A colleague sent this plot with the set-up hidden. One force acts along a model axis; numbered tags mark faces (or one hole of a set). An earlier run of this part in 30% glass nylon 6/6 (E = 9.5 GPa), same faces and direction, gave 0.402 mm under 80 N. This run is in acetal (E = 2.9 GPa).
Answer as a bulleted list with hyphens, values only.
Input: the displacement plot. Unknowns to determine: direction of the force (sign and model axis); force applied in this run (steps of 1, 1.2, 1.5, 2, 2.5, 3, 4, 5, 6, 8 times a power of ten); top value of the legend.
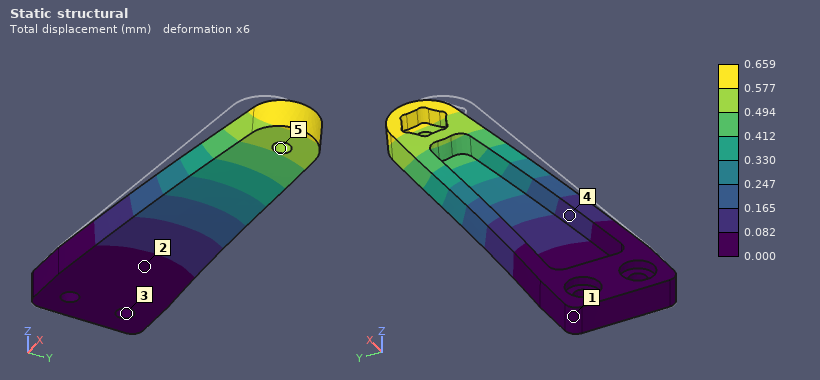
- +Y
- 40 N
- 0.659 mm
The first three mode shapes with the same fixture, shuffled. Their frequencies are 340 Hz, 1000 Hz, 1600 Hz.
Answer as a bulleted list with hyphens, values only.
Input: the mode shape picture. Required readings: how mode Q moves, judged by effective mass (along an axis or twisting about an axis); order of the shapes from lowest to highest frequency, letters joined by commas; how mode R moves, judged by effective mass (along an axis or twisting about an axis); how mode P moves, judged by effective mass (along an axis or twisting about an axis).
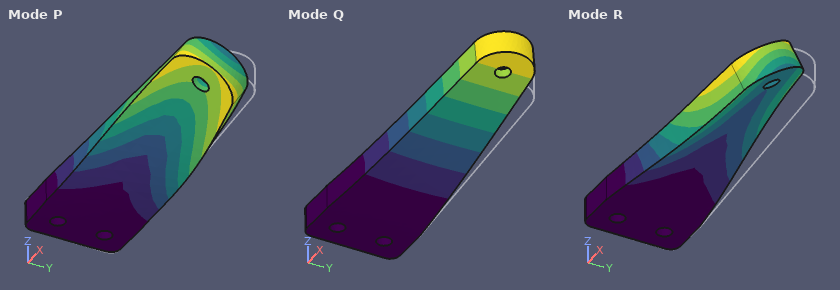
- along Z
- Q, R, P
- along Y
- along Y
